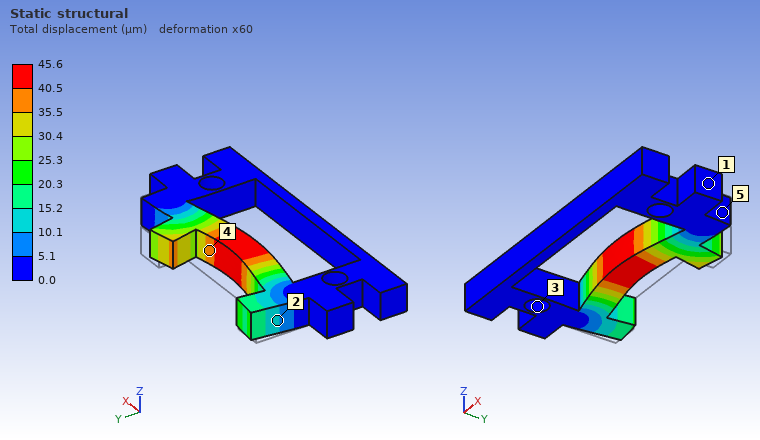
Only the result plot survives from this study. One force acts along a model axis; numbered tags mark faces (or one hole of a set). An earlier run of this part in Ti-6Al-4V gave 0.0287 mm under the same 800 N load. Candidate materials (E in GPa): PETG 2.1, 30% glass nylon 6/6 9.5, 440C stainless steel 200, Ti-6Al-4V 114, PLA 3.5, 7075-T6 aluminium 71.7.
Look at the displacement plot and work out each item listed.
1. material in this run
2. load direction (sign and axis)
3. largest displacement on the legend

7075-T6 aluminium
-Y
45.6 µm
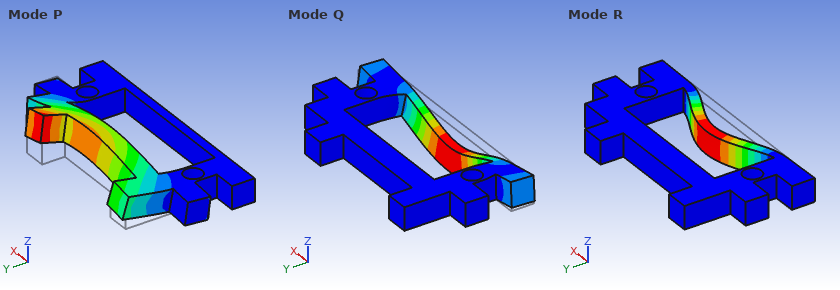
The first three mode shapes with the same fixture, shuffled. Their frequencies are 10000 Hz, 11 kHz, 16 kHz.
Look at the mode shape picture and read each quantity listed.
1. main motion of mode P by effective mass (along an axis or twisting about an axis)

along Z
